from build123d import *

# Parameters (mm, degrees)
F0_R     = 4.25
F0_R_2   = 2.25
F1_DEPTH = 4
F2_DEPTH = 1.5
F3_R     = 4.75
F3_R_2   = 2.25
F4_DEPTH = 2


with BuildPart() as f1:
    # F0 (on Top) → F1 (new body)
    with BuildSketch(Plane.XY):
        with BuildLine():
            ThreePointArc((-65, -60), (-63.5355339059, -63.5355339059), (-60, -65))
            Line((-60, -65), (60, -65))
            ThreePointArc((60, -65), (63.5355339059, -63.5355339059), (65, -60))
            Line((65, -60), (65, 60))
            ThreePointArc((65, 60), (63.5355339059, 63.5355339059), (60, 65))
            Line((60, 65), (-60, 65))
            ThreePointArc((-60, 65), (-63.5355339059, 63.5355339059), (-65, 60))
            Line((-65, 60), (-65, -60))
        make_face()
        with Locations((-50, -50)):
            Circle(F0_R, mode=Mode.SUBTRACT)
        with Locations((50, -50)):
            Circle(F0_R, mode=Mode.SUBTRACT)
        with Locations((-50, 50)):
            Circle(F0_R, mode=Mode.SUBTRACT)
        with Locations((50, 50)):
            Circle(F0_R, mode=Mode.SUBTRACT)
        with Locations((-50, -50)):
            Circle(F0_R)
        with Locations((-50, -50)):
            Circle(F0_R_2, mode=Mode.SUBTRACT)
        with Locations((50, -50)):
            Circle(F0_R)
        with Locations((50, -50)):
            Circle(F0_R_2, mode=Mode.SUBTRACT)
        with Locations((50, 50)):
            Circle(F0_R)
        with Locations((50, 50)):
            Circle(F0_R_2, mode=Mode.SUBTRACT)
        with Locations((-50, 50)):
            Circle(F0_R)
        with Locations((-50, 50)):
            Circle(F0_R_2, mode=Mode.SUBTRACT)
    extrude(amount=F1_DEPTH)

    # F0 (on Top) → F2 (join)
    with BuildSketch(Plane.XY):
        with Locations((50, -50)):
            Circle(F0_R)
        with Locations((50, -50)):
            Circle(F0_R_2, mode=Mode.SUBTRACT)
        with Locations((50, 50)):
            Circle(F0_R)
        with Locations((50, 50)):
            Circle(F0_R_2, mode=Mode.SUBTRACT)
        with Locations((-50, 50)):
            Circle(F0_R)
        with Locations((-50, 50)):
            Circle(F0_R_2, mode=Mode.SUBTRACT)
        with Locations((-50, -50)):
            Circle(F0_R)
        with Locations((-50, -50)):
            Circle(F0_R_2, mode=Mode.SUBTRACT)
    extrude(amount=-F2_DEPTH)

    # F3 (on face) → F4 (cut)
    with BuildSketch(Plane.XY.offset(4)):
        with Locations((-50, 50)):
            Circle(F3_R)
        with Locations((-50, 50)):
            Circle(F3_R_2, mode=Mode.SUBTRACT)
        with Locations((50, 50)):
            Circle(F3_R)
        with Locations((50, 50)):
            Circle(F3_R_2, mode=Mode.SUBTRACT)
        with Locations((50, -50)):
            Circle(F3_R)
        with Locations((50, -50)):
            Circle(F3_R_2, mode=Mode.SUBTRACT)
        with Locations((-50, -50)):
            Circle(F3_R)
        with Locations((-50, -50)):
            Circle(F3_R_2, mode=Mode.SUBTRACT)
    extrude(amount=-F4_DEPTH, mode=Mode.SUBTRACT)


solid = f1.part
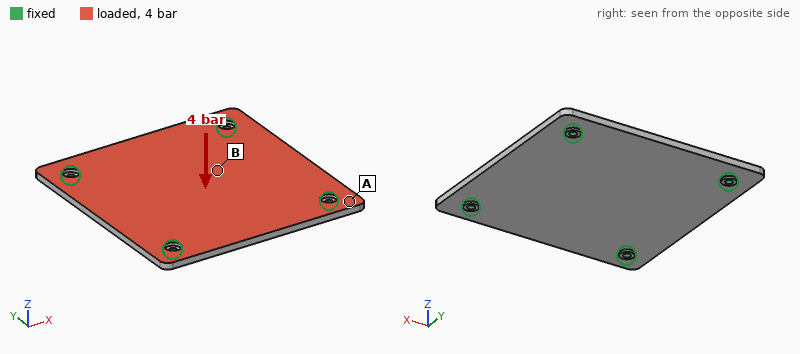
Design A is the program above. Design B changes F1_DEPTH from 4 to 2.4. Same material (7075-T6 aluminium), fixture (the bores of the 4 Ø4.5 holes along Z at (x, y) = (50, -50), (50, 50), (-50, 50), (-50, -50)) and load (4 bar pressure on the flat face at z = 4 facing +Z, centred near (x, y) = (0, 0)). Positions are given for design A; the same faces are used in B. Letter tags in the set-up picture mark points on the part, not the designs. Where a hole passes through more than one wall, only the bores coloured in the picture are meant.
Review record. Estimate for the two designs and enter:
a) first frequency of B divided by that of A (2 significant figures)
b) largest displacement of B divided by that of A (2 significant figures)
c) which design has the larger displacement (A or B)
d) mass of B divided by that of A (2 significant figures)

0.68
3.7
B
0.60
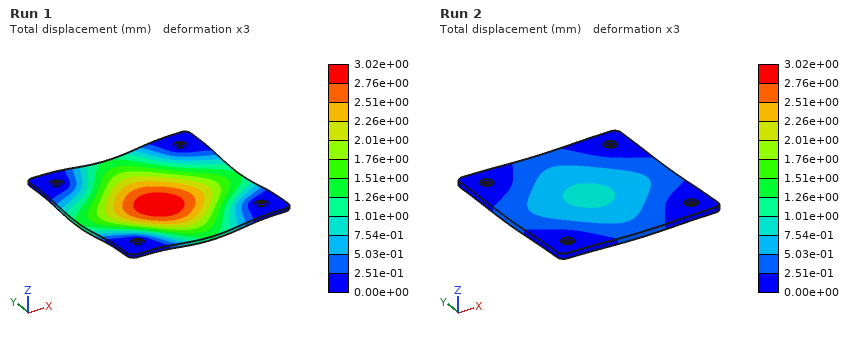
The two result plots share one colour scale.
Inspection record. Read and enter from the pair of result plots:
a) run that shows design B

Run 1
